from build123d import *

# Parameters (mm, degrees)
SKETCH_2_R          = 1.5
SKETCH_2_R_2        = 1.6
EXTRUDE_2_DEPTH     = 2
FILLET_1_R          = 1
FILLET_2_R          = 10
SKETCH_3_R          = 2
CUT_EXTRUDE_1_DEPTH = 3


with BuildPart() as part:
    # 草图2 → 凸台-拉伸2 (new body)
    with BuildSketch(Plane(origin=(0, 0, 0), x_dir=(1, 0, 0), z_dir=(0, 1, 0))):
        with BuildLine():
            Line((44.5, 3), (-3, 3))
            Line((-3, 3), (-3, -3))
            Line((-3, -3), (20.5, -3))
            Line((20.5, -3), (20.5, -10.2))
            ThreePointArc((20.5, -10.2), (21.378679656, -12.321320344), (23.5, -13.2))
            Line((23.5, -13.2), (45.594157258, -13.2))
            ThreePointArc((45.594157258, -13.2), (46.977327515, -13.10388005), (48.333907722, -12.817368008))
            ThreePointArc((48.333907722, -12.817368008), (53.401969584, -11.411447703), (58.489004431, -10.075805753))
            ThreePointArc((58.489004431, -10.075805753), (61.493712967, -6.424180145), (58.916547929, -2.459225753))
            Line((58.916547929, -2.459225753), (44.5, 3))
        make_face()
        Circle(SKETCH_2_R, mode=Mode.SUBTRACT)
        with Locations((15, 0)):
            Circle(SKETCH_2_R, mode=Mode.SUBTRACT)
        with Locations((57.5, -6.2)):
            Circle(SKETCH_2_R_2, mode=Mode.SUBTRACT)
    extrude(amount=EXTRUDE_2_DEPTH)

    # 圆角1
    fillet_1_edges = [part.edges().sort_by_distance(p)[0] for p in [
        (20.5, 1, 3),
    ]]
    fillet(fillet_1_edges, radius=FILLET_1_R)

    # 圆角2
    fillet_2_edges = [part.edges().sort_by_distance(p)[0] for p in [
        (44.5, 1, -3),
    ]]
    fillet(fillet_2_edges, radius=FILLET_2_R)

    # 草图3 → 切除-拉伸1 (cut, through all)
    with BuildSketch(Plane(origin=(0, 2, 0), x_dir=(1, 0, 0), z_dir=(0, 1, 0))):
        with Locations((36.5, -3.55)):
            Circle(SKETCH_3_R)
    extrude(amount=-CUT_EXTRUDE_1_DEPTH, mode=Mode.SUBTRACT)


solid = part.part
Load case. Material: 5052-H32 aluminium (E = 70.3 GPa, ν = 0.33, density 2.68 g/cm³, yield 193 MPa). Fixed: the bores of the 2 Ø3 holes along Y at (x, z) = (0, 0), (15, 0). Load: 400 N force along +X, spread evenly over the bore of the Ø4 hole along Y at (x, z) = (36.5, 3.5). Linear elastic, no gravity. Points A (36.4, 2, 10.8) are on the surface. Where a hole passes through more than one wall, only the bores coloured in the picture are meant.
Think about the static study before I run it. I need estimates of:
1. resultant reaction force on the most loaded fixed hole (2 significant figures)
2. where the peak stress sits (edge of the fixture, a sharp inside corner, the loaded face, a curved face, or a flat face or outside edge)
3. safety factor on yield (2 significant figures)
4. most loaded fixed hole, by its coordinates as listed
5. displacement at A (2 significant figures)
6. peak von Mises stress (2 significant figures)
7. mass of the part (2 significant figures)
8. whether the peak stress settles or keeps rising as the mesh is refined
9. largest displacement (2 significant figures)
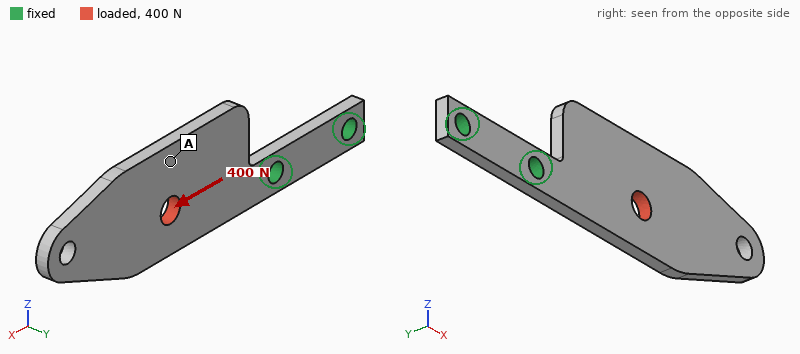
390 N
a curved face
0.69
(15, 0)
0.099 mm
280 MPa
3.7 g
settles
0.20 mm
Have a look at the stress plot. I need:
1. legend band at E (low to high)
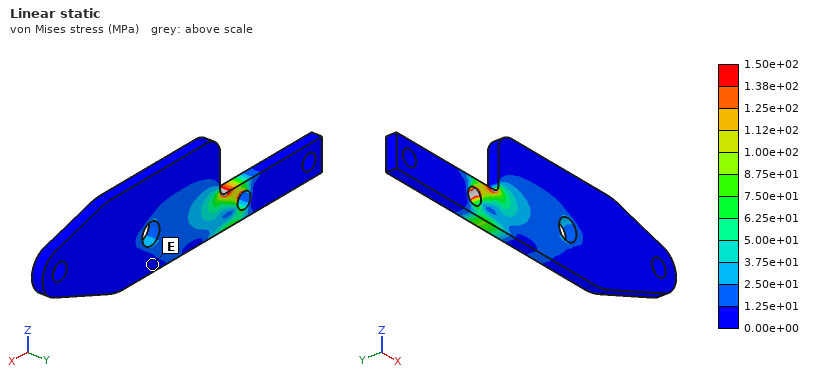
0.00e+00 to 1.25e+01 MPa
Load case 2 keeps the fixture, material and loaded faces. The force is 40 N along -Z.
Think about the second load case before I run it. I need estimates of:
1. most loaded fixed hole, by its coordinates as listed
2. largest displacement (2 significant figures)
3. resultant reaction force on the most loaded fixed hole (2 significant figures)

(15, 0)
0.11 mm
50 N
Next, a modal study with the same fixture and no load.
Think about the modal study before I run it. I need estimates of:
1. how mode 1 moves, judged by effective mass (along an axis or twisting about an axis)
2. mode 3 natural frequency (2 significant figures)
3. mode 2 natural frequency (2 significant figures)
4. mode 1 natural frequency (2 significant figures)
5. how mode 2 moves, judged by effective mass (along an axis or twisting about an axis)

along Y
3400 Hz
2100 Hz
710 Hz
along Z
